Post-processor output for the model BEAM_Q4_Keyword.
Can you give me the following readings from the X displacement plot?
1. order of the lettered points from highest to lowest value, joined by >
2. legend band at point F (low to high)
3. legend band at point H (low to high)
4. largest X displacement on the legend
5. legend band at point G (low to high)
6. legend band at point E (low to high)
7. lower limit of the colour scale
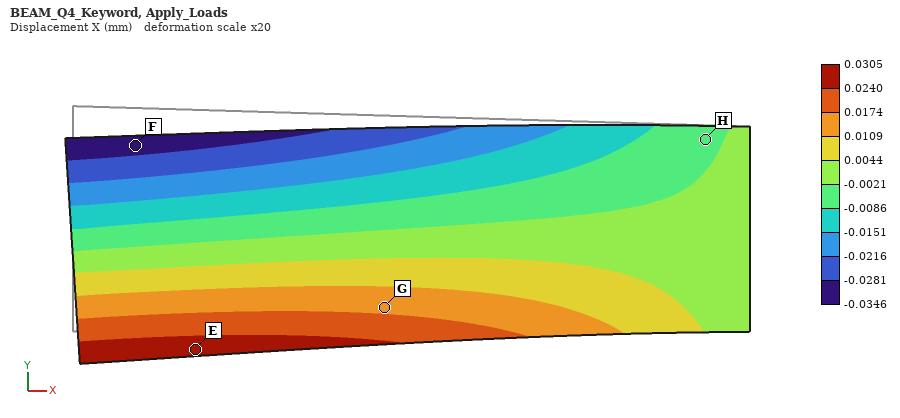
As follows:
E > G > H > F
-0.0346 to -0.0281 mm
-0.0086 to -0.0021 mm
0.0305 mm
0.0109 to 0.0174 mm
0.0240 to 0.0305 mm
-0.0346 mm
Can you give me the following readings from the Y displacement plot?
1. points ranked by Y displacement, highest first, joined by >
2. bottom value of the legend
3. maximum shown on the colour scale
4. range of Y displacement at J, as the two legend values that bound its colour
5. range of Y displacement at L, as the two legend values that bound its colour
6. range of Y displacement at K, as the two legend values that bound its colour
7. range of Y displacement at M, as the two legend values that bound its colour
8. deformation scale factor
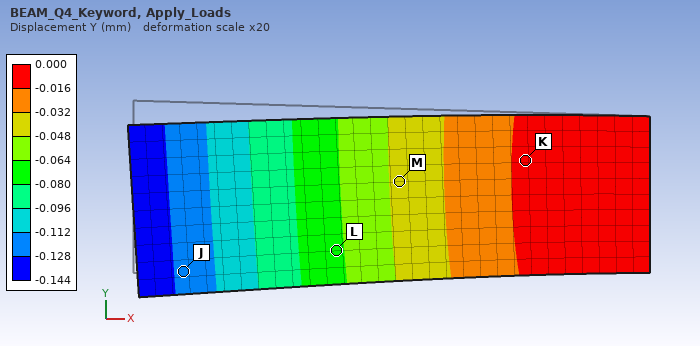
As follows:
K > M > L > J
-0.144 mm
0.000 mm
-0.128 to -0.112 mm
-0.080 to -0.064 mm
-0.016 to 0.000 mm
-0.048 to -0.032 mm
20
